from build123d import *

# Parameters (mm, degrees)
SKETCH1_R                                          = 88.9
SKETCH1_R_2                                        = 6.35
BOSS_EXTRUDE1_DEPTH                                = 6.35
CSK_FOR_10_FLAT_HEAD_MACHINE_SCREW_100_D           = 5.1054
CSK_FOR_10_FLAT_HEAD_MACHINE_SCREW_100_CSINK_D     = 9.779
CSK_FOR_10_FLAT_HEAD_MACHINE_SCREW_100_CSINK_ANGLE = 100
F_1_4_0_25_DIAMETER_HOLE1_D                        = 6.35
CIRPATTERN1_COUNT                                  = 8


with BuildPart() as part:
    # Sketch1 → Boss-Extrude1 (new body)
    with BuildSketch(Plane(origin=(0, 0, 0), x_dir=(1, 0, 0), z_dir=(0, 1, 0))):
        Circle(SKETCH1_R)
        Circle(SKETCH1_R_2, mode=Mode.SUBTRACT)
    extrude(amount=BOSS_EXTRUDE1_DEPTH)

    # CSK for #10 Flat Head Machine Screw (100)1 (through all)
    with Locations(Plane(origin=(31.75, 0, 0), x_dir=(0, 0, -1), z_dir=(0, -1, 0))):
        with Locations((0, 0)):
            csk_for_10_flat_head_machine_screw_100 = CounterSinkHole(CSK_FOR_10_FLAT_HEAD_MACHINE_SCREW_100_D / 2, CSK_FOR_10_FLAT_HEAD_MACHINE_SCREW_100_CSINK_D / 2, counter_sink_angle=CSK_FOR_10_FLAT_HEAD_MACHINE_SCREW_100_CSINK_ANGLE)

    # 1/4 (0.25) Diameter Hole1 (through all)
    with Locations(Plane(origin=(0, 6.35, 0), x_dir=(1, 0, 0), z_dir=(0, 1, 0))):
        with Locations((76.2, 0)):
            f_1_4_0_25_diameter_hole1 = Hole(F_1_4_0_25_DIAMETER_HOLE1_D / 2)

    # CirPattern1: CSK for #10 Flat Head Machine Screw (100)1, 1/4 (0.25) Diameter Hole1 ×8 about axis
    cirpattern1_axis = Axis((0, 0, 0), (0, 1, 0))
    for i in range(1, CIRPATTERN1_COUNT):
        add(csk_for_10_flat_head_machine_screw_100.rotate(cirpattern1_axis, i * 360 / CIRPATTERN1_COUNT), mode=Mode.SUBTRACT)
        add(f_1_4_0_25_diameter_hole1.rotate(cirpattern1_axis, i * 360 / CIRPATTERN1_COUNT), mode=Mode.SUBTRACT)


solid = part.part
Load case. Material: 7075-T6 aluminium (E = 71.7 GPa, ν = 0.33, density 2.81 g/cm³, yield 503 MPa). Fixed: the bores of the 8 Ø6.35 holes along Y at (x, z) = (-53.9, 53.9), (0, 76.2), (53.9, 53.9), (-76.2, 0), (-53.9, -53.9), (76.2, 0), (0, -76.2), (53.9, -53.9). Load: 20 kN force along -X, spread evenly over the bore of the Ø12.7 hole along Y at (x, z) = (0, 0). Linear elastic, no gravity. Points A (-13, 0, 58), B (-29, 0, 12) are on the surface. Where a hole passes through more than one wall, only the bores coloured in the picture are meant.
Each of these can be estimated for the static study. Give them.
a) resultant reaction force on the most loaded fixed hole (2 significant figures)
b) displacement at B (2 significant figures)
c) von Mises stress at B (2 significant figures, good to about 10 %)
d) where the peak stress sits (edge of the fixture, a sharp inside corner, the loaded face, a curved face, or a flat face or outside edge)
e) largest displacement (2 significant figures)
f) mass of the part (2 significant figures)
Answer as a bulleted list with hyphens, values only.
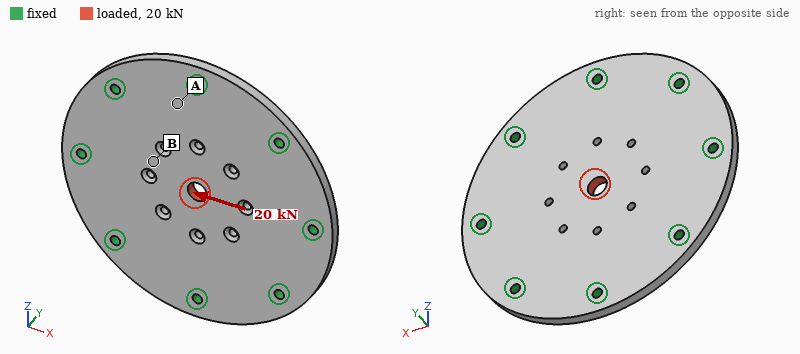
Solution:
- 4.1 kN
- 16 µm
- 28 MPa
- the loaded face
- 34 µm
- 430 g
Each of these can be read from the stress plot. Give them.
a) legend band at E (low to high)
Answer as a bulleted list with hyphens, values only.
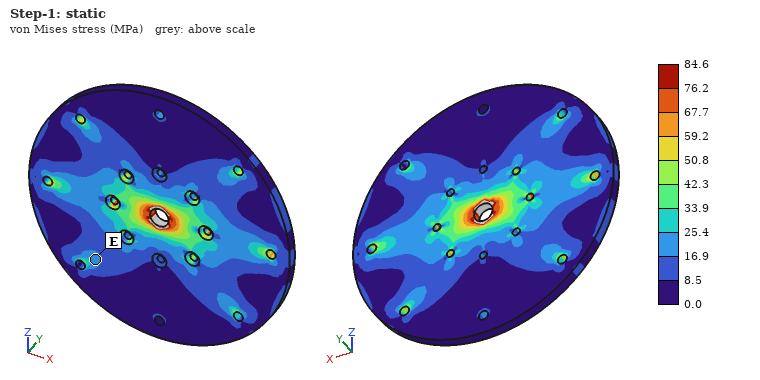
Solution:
- 16.9 to 25.4 MPa
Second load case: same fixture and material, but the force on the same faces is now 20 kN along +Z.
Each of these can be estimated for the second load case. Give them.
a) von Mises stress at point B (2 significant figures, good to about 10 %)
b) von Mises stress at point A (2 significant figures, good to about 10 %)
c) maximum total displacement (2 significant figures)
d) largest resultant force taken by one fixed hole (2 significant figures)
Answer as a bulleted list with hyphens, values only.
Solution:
- 17 MPa
- 15 MPa
- 34 µm
- 4.1 kN
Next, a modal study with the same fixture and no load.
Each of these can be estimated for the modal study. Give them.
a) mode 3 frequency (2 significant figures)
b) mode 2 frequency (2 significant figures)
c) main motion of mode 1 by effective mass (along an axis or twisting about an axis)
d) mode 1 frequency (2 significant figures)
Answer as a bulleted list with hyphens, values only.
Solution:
- 4800 Hz
- 4800 Hz
- along Y
- 2400 Hz
